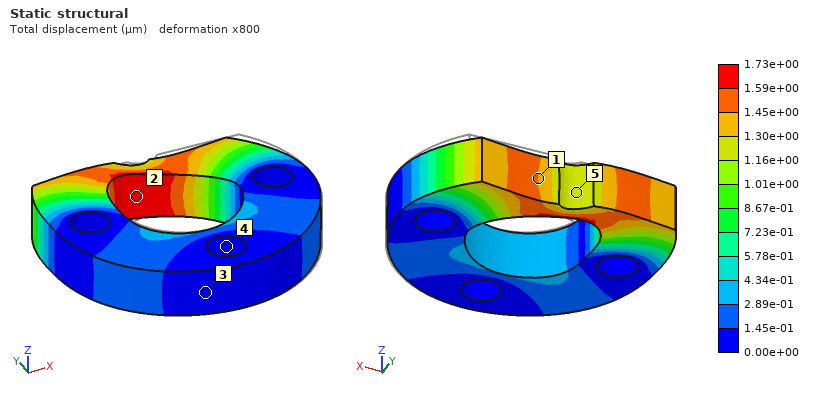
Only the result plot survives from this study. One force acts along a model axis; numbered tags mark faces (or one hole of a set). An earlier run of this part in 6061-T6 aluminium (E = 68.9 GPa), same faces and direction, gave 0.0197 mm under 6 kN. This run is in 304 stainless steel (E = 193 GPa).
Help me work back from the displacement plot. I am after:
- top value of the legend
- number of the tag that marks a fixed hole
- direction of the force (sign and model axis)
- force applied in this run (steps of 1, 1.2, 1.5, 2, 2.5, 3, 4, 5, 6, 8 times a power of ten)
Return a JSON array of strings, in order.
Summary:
["1.73e+00 µm", "4", "-X", "1.5 kN"]
